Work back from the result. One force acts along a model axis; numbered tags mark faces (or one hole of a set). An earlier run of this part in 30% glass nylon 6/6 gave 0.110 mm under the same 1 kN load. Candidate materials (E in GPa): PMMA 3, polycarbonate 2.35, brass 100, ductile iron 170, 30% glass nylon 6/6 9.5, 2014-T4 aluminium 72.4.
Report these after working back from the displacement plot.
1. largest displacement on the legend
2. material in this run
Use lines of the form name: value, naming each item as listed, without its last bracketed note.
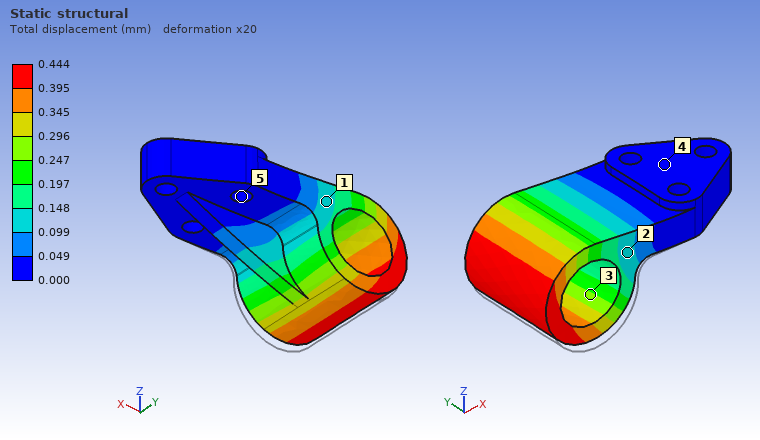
largest displacement on the legend: 0.444 mm
material in this run: polycarbonate
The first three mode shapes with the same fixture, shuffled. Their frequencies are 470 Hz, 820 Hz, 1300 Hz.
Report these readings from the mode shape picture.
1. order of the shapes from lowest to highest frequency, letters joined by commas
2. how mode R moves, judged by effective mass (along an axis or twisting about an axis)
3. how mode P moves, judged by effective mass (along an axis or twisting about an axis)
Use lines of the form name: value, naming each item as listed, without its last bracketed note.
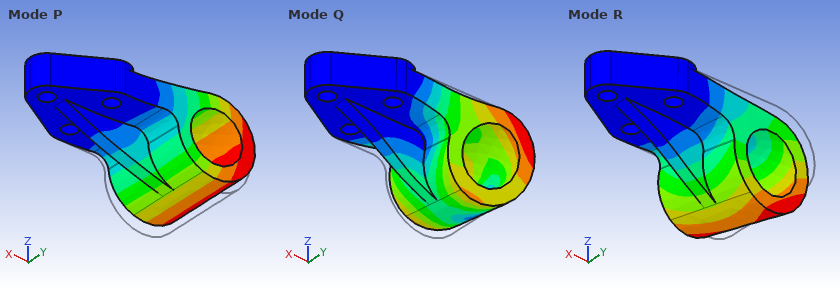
order of the shapes from lowest to highest frequency, letters joined by commas: P, R, Q
how mode R moves, judged by effective mass: along Y
how mode P moves, judged by effective mass: along Z
